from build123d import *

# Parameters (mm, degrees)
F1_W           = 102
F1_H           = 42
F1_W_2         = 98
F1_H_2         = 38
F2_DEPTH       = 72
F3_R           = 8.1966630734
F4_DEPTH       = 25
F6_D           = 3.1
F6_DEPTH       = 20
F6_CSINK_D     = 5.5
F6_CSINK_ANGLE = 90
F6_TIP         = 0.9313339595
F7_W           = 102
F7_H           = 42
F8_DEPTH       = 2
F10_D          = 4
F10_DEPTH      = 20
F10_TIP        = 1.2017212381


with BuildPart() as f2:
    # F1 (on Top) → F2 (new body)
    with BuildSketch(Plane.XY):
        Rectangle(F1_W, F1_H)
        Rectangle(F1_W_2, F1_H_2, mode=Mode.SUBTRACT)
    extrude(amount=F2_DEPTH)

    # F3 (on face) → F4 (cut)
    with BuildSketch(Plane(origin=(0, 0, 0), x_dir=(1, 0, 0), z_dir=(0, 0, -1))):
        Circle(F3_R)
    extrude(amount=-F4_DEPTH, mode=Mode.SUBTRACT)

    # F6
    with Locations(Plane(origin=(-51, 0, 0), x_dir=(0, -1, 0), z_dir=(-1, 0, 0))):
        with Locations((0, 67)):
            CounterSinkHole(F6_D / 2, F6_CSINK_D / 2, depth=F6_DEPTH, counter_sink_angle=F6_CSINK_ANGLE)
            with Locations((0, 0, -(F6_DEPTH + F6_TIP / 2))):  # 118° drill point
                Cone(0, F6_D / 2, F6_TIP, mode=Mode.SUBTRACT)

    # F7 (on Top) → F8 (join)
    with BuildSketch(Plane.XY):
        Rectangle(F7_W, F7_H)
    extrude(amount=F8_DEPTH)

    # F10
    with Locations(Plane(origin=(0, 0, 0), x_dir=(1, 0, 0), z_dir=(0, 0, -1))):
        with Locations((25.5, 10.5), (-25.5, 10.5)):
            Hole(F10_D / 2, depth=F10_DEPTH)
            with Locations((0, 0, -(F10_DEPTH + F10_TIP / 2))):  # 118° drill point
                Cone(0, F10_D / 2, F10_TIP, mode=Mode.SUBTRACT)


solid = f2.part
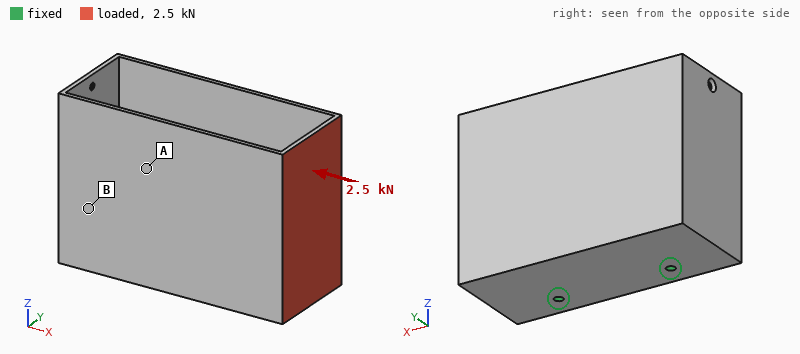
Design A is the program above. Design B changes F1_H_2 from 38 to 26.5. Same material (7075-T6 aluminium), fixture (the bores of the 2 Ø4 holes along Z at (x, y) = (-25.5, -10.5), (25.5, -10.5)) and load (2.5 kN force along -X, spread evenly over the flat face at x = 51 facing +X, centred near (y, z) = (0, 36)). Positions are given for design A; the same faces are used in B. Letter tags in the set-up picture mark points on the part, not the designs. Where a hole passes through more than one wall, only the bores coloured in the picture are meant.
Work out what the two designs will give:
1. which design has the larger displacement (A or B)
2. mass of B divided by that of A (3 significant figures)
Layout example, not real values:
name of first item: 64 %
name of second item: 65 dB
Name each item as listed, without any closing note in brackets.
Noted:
which design has the larger displacement: A
mass of B divided by that of A: 2.65
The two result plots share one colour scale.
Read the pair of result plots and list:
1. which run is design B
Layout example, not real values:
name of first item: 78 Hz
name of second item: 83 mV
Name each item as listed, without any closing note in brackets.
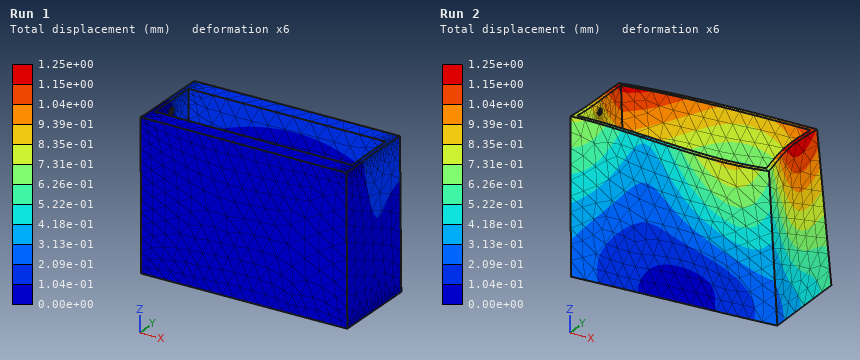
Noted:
which run is design B: Run 1
